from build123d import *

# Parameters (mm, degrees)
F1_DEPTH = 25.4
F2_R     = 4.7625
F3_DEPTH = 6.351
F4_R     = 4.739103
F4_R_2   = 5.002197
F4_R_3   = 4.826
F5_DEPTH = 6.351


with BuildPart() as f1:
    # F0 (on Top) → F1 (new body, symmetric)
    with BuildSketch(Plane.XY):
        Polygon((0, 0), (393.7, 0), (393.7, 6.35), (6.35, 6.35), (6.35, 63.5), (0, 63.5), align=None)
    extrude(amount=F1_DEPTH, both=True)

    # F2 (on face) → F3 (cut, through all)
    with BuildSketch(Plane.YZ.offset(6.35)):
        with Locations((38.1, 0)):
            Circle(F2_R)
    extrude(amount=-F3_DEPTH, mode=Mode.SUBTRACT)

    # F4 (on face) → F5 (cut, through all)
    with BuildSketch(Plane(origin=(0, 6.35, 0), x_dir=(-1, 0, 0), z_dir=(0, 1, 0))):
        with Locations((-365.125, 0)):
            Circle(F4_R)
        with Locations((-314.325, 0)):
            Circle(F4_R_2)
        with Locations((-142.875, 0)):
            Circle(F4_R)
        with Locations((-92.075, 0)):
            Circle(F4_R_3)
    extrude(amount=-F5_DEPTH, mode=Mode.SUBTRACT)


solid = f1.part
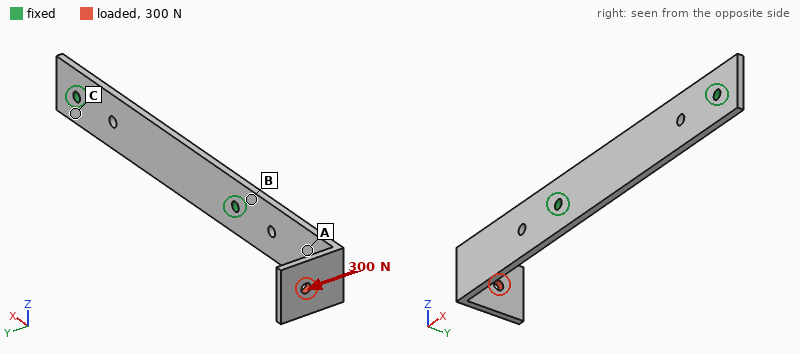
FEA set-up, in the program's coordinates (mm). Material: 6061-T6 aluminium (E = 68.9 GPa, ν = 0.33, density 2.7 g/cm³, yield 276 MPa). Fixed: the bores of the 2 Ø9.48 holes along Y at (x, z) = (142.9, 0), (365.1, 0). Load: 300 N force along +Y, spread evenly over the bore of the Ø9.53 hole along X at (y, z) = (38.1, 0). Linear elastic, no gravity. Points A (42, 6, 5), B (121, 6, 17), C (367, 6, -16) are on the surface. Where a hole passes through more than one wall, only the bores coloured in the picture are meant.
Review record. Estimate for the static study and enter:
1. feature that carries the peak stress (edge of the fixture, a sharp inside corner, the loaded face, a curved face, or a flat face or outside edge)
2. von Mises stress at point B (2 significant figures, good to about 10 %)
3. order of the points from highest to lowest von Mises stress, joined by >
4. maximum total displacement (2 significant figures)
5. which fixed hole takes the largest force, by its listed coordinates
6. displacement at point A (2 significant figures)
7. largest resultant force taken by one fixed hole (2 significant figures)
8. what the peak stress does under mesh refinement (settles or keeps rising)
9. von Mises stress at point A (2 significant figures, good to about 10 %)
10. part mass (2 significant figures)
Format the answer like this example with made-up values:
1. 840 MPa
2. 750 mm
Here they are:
1. edge of the fixture
2. 100 MPa
3. B > A > C
4. 4.5 mm
5. (142.9, 0)
6. 2.1 mm
7. 300 N
8. keeps rising
9. 34 MPa
10. 390 g
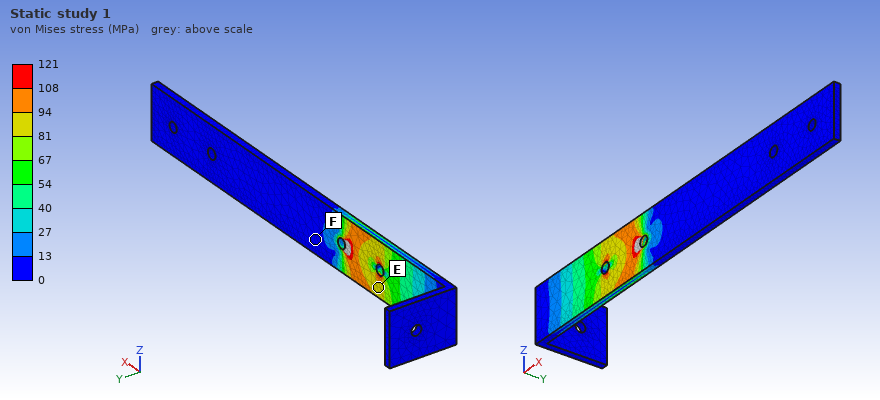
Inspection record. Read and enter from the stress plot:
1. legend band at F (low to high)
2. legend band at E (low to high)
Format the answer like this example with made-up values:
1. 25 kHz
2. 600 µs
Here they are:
1. 0 to 13 MPa
2. 81 to 94 MPa
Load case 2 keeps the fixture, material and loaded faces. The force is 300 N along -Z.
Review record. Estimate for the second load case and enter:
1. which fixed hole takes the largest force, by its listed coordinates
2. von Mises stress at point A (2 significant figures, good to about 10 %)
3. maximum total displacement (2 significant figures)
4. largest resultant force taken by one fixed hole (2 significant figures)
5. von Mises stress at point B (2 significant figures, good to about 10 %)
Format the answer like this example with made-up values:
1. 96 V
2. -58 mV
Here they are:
1. (142.9, 0)
2. 30 MPa
3. 0.99 mm
4. 430 N
5. 25 MPa
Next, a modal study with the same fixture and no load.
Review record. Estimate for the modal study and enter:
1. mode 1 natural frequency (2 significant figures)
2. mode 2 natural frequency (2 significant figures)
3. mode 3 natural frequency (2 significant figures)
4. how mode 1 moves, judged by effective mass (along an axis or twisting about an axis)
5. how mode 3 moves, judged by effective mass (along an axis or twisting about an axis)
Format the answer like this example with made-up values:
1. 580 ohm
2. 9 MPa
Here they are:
1. 150 Hz
2. 460 Hz
3. 680 Hz
4. along Y
5. along Y
